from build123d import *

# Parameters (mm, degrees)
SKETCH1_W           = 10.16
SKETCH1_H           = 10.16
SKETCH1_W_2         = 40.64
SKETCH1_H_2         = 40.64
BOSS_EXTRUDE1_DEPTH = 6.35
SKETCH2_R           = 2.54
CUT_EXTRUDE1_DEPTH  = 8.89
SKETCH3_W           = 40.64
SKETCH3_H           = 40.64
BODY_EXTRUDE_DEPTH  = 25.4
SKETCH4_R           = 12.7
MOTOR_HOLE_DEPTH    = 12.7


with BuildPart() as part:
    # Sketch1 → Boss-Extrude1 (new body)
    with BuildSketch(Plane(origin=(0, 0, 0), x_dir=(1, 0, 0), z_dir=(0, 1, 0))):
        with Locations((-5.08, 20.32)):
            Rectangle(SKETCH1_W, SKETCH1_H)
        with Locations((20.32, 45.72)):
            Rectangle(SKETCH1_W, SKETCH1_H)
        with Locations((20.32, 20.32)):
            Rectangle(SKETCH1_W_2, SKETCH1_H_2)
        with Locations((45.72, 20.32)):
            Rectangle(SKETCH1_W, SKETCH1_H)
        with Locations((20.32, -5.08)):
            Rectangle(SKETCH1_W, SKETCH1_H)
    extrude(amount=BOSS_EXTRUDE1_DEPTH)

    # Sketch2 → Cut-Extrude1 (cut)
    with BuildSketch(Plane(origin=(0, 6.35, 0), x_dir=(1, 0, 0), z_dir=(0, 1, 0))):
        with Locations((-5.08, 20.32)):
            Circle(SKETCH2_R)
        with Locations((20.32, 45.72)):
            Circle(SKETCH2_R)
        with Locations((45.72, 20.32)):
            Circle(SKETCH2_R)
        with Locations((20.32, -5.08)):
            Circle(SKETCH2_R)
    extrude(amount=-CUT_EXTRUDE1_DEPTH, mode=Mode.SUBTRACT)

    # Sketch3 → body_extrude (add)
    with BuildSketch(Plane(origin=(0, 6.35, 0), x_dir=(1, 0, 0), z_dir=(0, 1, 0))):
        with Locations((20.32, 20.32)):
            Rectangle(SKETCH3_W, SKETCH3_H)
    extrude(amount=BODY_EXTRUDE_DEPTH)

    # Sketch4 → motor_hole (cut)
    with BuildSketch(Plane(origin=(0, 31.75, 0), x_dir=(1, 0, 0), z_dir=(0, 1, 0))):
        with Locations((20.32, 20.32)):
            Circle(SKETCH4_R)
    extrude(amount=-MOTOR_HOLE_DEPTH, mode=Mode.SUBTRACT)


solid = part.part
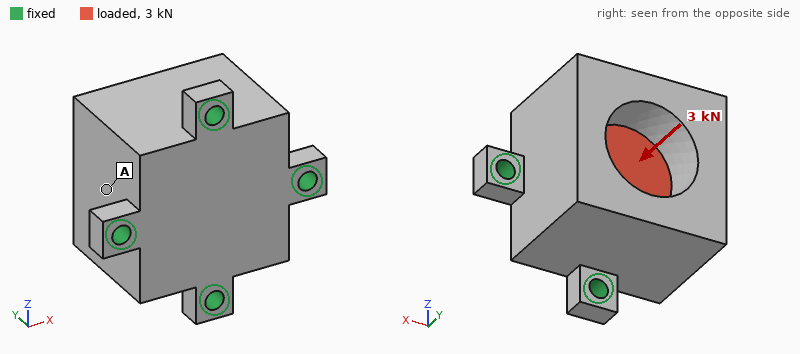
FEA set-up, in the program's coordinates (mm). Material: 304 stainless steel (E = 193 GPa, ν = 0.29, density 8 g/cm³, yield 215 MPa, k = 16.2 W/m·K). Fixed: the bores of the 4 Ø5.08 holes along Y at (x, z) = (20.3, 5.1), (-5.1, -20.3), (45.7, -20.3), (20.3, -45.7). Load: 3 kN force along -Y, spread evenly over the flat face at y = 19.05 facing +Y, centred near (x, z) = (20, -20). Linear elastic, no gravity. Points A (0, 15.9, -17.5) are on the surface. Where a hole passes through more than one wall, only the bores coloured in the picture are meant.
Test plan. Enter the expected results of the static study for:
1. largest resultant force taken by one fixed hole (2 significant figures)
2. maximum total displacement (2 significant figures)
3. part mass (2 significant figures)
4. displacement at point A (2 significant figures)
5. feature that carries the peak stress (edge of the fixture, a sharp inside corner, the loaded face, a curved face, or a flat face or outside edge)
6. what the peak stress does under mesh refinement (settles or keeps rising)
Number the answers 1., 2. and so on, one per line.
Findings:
1. 820 N
2. 2.0 µm
3. 380 g
4. 1.4 µm
5. edge of the fixture
6. keeps rising
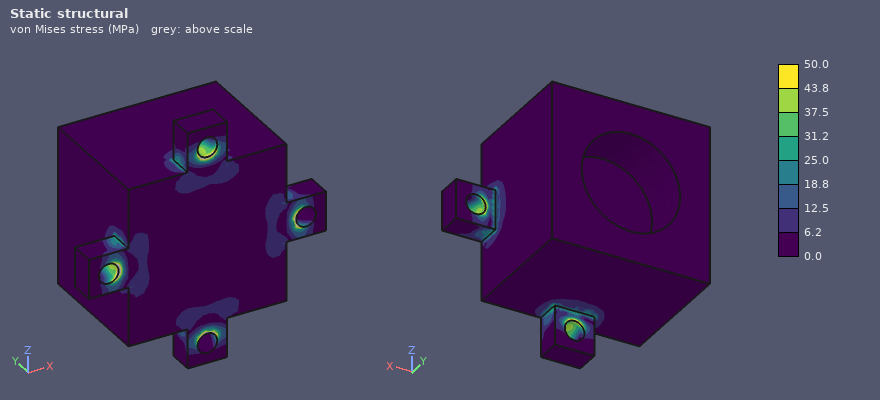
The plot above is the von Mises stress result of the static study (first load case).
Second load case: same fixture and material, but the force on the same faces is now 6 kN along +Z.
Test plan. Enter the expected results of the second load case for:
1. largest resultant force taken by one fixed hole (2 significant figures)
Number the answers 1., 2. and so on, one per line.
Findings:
1. 3.1 kN
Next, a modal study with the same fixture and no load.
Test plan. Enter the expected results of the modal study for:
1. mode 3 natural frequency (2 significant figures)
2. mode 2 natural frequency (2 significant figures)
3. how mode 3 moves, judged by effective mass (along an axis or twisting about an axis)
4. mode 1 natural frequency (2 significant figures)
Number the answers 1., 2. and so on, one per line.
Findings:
1. 12 kHz
2. 8900 Hz
3. along Y
4. 8900 Hz
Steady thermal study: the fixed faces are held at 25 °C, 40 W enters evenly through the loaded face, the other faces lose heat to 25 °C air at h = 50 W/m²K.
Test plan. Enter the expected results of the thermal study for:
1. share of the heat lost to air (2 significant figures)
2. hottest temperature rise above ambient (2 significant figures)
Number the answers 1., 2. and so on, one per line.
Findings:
1. 43 %
2. 80 K
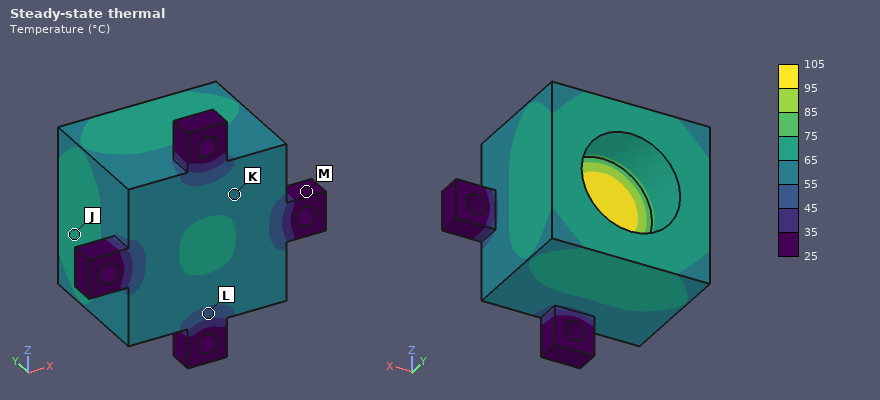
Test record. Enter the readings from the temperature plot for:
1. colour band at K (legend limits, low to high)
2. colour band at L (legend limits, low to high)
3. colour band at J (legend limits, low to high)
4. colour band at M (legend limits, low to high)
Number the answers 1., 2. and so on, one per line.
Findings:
1. 55 to 65 °C
2. 45 to 55 °C
3. 65 to 75 °C
4. 25 to 35 °C
